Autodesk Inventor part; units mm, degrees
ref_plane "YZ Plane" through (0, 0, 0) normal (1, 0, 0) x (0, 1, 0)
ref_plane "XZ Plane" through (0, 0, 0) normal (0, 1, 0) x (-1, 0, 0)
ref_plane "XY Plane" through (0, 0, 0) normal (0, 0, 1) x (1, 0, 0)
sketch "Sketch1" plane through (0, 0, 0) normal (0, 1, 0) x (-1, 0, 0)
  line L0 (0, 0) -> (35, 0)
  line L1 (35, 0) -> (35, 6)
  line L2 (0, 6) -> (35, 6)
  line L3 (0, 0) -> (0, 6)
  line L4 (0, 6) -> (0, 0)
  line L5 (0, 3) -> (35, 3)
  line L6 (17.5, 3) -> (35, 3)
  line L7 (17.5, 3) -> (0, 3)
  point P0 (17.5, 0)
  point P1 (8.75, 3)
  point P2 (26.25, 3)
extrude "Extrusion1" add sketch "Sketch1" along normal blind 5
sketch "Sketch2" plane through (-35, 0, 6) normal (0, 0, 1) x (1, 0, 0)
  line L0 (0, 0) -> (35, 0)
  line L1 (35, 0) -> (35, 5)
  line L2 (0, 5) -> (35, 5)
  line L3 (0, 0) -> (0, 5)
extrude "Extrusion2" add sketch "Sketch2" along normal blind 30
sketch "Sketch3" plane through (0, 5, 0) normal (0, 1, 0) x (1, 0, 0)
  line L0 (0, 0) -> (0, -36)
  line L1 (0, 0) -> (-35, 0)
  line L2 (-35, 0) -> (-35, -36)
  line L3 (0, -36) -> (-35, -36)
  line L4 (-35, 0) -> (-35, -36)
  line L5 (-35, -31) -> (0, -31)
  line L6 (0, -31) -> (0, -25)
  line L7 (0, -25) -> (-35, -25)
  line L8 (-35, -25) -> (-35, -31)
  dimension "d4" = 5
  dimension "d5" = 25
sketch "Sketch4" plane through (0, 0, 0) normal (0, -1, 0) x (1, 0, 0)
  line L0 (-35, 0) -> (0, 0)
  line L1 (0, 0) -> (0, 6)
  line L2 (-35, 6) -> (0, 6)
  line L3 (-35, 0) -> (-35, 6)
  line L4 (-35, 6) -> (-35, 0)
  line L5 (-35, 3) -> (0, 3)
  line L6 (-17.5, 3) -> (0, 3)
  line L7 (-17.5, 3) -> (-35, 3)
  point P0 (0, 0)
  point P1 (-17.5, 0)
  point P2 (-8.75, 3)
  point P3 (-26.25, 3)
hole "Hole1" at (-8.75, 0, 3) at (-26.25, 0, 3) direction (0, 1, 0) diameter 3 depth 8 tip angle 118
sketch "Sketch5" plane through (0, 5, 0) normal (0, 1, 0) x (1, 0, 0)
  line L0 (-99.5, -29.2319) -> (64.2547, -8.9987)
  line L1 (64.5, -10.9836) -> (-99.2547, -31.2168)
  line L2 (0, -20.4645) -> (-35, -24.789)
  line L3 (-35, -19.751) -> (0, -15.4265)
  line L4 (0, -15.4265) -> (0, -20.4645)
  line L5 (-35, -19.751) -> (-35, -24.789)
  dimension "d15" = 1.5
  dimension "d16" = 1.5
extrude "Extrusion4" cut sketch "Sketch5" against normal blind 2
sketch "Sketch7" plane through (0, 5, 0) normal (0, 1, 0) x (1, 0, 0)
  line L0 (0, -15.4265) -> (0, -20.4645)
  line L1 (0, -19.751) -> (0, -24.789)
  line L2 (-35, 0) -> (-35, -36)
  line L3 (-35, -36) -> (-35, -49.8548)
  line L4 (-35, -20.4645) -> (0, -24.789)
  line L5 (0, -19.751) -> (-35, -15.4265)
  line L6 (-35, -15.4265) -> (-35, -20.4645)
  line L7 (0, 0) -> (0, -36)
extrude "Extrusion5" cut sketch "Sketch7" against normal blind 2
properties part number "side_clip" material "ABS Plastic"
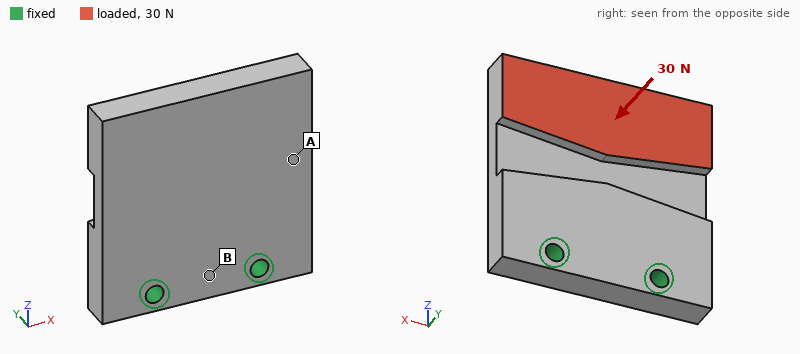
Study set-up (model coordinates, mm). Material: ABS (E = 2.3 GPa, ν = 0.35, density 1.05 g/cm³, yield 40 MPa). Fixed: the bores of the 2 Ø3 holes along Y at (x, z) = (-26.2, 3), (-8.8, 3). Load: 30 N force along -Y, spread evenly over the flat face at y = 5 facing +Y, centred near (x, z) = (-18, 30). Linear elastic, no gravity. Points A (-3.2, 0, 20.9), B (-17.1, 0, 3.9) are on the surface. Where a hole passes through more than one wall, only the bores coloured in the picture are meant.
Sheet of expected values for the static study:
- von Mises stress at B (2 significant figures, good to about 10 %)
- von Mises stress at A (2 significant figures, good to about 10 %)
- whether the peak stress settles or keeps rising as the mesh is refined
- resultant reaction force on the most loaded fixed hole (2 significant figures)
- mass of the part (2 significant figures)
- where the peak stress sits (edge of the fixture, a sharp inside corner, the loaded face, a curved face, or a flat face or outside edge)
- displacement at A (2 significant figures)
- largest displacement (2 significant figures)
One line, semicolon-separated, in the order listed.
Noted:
1.7 MPa; 4.6 MPa; keeps rising; 15 N; 6.0 g; edge of the fixture; 0.17 mm; 0.54 mm
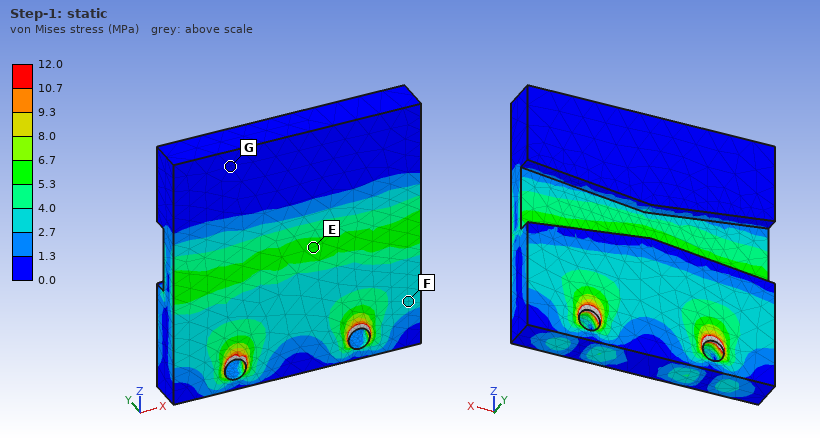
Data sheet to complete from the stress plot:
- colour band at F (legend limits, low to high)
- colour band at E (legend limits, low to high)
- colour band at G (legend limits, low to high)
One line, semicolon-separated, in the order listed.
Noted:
2.7 to 4.0 MPa; 5.3 to 6.7 MPa; 0.0 to 1.3 MPa
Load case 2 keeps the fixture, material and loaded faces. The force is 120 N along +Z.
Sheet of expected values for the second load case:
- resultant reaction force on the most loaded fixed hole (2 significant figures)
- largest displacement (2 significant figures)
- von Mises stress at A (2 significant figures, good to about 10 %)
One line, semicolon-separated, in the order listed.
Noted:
60 N; 0.47 mm; 5.9 MPa
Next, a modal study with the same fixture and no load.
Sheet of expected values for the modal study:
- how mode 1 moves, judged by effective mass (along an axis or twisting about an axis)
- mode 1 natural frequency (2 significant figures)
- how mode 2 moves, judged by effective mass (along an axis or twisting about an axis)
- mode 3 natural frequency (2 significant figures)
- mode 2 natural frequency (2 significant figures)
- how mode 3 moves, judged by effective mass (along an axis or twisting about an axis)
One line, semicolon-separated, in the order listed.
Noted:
along Y; 880 Hz; twisting about Z; 3500 Hz; 2000 Hz; along X
